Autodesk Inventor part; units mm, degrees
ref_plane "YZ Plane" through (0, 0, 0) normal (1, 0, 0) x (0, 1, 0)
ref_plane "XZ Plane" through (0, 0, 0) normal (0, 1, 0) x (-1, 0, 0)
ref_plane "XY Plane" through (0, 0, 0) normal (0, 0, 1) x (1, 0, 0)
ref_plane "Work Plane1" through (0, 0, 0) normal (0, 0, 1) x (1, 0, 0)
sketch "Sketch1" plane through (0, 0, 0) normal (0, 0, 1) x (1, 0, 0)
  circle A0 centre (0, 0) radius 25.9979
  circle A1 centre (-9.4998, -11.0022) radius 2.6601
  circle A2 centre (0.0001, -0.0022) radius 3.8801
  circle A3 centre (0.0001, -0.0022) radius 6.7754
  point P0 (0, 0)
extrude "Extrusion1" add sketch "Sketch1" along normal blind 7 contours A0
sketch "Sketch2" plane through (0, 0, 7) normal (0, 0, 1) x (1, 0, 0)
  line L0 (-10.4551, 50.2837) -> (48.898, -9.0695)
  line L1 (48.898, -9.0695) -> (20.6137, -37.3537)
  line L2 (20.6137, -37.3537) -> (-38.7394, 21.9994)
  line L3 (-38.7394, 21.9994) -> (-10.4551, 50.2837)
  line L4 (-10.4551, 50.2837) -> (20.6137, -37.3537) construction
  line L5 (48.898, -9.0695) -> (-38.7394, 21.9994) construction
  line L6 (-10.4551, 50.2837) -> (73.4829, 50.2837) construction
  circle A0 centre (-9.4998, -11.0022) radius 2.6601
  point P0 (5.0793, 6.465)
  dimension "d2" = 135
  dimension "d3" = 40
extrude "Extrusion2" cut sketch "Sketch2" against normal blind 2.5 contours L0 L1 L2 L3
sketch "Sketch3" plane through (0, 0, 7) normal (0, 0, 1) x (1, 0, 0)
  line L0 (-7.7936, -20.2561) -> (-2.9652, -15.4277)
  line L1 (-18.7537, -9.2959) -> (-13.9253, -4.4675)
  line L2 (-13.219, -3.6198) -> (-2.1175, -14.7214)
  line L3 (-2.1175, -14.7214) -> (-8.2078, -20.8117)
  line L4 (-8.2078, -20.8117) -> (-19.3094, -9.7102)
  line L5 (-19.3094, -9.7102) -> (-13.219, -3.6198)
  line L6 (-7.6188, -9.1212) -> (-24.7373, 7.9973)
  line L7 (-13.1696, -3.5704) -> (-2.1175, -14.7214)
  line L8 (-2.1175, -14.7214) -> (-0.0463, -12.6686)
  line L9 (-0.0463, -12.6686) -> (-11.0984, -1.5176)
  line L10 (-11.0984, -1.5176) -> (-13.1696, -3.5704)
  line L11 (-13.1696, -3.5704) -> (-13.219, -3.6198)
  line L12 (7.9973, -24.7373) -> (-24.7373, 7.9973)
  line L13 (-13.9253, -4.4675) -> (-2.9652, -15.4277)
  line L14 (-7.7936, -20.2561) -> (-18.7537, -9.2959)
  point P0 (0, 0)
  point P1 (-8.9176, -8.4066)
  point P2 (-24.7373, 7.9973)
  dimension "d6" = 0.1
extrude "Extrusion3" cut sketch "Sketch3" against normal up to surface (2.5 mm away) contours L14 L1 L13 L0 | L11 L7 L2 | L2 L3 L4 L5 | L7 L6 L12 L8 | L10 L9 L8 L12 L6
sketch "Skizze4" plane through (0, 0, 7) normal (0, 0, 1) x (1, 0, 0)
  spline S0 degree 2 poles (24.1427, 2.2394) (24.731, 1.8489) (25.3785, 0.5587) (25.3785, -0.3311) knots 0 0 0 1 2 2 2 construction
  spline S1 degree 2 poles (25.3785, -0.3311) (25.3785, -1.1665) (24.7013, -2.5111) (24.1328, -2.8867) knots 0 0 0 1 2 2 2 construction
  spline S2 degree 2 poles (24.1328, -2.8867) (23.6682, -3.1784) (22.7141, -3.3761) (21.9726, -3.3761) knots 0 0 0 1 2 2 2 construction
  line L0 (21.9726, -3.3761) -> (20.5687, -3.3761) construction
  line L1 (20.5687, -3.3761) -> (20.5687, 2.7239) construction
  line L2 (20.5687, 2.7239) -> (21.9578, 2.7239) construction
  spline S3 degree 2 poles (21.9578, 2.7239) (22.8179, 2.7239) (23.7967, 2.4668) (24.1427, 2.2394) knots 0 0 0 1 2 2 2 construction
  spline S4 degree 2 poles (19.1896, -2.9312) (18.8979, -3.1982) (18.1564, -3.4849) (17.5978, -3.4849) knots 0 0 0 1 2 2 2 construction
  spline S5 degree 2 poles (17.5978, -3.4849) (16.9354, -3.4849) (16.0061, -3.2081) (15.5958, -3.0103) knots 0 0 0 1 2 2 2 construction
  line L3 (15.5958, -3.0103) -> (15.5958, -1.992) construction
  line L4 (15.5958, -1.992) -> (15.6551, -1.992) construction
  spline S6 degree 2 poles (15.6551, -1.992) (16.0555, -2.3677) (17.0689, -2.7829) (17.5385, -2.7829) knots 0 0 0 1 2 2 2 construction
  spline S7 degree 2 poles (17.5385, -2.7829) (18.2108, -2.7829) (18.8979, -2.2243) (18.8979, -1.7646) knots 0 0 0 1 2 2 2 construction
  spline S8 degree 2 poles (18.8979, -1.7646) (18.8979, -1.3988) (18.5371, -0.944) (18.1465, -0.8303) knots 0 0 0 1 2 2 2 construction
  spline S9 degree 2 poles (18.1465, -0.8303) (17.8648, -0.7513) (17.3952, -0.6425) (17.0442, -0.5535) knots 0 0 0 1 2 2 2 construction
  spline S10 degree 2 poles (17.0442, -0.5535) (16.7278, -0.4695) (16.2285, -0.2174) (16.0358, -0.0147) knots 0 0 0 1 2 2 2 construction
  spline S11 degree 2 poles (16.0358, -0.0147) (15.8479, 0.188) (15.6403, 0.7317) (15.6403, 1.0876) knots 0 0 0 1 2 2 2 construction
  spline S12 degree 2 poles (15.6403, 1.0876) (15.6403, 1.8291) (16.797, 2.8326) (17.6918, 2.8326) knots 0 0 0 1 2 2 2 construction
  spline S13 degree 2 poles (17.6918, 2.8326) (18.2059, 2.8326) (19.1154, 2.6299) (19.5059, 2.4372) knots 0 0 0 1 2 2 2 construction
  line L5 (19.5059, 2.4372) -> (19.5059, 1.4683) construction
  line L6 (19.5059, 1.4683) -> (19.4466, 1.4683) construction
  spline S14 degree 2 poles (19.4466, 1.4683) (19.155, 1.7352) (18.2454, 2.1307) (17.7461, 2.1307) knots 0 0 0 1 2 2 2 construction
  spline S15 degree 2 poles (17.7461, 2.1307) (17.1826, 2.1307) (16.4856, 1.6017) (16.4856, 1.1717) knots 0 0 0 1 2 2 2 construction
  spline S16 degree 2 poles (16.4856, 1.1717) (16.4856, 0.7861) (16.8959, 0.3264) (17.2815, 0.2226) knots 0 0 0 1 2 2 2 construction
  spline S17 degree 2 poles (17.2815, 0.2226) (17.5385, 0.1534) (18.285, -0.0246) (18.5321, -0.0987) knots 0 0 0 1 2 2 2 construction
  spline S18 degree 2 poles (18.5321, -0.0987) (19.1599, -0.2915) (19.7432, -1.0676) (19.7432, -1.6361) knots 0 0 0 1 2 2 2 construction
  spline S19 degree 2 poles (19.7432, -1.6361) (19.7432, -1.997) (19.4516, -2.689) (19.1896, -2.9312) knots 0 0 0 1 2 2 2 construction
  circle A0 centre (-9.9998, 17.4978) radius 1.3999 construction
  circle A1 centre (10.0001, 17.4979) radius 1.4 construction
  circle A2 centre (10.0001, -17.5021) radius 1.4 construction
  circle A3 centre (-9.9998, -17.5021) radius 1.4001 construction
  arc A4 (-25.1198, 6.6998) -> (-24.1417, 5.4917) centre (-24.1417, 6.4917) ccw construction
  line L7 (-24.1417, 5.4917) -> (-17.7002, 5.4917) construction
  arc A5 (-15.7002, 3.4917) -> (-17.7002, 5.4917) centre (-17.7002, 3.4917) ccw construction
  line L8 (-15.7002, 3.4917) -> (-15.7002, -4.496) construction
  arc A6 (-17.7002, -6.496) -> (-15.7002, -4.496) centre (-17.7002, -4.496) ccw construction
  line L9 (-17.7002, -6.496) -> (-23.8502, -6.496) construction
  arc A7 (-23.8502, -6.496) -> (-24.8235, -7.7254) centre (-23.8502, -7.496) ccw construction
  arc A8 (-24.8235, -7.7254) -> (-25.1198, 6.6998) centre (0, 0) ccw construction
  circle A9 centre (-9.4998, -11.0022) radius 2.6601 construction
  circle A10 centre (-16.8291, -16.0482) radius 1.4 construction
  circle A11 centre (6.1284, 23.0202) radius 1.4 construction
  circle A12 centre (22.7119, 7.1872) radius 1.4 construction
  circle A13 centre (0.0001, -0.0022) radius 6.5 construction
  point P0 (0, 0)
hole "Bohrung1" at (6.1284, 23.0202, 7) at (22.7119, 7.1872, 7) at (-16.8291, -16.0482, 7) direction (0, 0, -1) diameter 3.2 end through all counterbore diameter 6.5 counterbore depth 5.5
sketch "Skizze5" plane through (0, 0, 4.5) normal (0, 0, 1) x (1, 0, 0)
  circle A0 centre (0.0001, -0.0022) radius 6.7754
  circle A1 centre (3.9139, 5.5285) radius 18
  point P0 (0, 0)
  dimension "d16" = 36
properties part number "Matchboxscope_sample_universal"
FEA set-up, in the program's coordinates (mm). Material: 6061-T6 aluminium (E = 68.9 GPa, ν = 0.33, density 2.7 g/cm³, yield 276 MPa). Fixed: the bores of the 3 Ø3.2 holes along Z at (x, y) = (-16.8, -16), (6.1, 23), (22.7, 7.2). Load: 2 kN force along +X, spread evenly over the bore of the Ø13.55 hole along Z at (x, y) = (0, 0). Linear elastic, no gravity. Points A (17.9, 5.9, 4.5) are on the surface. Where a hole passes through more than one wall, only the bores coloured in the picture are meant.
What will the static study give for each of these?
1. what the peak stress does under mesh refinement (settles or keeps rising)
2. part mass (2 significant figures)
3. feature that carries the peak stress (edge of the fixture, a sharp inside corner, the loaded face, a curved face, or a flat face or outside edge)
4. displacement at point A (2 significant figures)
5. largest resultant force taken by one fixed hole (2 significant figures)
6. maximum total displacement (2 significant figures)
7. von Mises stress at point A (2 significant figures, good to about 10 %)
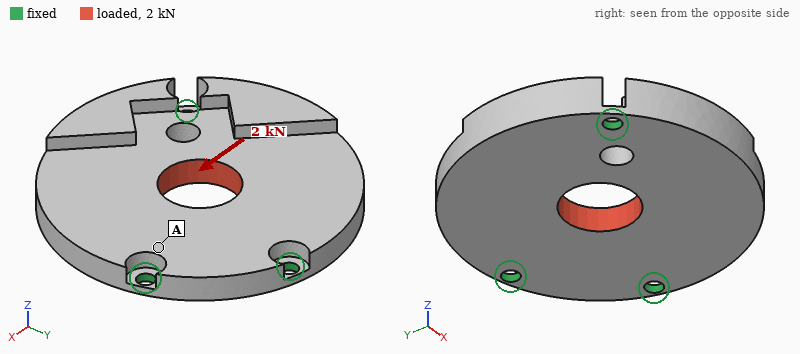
keeps rising
25 g
edge of the fixture
5.0 µm
780 N
21 µm
14 MPa
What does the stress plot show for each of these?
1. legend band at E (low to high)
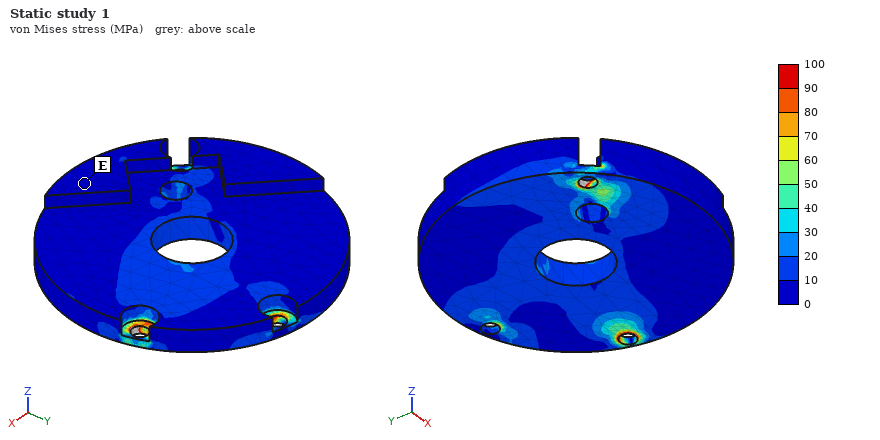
0 to 10 MPa
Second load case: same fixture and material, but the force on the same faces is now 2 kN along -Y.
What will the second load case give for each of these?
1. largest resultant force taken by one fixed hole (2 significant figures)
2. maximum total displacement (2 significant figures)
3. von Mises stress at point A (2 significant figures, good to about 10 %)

770 N
23 µm
13 MPa
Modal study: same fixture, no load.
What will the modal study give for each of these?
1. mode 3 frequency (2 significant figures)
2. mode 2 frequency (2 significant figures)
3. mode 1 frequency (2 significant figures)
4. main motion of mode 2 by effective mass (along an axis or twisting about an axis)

12 kHz
5100 Hz
3800 Hz
along Z
